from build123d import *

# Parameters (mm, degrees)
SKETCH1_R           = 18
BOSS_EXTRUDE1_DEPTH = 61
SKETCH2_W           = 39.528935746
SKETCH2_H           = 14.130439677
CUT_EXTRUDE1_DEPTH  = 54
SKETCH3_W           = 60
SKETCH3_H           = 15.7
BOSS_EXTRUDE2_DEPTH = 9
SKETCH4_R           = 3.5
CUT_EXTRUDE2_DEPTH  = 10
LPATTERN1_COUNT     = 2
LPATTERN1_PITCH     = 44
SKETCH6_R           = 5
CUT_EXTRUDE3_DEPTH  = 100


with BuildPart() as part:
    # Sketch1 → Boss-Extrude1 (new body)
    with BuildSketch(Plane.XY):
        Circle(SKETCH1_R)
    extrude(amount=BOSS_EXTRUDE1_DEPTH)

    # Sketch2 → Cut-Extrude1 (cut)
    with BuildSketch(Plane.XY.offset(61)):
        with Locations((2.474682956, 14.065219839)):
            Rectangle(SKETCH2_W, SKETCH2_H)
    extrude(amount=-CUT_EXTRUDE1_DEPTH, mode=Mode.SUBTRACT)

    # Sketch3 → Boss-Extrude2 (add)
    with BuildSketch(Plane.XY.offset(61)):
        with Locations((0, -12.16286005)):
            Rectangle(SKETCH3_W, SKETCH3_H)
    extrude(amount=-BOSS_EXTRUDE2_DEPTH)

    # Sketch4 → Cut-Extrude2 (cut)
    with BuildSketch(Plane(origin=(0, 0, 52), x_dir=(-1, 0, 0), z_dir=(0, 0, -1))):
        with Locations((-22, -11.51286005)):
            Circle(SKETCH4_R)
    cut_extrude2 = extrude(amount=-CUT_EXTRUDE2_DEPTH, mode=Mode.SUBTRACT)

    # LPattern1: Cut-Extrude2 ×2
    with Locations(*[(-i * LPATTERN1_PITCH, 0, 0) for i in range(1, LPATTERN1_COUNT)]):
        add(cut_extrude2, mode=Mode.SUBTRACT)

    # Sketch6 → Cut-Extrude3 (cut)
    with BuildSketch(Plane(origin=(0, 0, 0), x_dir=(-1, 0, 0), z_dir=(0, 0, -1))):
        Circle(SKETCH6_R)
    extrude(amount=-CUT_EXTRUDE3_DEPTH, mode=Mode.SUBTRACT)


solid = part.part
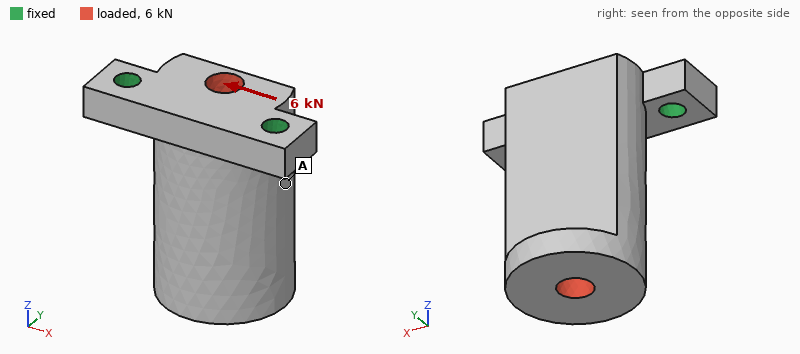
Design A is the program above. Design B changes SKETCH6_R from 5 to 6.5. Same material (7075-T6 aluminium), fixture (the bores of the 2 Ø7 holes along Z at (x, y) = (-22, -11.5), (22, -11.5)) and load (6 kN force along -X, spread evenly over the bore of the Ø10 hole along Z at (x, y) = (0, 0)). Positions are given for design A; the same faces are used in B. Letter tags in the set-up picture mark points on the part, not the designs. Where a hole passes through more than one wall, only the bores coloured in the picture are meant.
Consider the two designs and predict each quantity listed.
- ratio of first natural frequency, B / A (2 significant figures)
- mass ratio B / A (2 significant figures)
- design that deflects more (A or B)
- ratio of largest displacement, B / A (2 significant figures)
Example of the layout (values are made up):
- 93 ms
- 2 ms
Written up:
- 1.0
- 0.93
- B
- 1.1
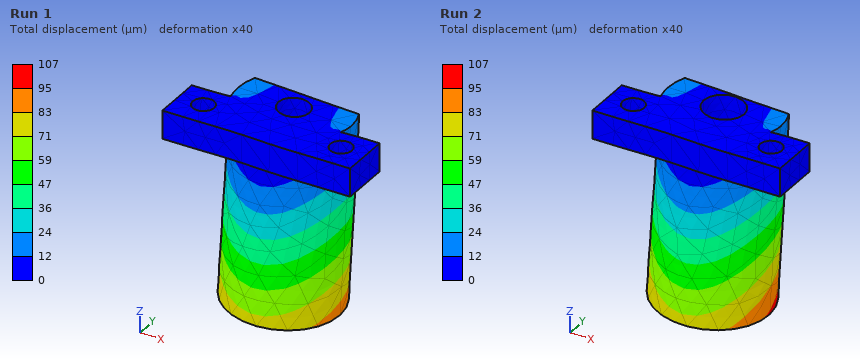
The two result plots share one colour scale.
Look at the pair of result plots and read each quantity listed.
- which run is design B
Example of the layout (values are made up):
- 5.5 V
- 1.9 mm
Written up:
- Run 2
